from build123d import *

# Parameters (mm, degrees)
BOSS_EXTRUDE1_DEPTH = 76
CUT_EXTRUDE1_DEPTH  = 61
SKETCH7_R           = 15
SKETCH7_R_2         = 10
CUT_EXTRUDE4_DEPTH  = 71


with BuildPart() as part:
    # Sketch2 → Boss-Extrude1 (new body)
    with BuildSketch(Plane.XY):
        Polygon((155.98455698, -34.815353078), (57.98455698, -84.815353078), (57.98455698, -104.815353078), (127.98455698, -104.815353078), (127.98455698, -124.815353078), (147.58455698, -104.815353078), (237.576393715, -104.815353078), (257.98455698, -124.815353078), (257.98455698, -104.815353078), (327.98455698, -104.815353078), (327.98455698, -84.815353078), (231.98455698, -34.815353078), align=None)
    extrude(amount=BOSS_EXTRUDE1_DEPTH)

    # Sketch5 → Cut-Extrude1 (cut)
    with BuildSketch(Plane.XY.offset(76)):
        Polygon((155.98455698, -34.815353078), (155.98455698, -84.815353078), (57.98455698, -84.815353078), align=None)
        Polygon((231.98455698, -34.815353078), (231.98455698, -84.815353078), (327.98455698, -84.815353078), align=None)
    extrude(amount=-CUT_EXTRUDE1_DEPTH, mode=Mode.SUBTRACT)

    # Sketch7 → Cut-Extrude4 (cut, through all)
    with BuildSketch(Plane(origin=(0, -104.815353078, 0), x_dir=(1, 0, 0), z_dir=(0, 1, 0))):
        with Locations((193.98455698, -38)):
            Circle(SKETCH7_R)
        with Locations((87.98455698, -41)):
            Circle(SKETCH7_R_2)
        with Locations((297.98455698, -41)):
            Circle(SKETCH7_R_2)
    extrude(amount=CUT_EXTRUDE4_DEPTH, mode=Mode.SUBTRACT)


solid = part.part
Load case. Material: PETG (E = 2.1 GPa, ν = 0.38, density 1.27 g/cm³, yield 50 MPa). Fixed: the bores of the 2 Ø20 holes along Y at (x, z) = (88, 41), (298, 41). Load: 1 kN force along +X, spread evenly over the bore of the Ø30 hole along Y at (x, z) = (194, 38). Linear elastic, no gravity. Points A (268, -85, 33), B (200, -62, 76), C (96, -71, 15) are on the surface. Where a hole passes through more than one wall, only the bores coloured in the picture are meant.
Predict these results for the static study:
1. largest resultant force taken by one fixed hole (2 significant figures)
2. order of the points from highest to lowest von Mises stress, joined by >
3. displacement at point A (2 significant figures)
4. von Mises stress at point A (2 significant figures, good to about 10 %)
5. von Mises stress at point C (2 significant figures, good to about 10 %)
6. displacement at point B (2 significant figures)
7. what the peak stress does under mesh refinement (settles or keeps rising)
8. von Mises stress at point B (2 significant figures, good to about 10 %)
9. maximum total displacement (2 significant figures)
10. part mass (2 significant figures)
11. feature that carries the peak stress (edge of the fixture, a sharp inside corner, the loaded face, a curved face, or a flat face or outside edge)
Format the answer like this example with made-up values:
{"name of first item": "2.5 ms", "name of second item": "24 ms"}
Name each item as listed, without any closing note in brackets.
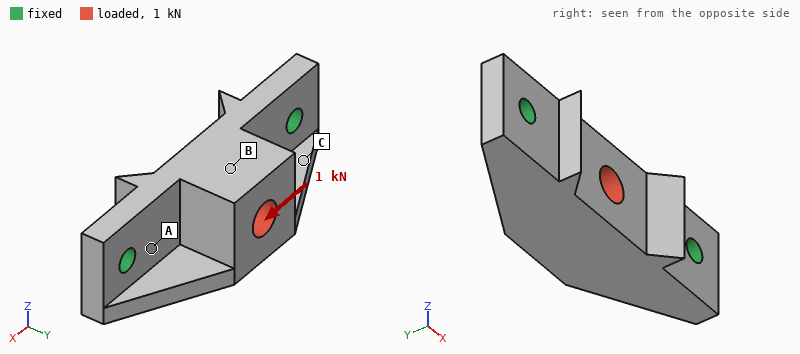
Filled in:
{"largest resultant force taken by one fixed hole": "520 N", "order of the points from highest to lowest von Mises stress, joined by >": "A > C > B", "displacement at point A": "7.8 µm", "von Mises stress at point A": "0.52 MPa", "von Mises stress at point C": "0.34 MPa", "displacement at point B": "28 µm", "what the peak stress does under mesh refinement": "keeps rising", "von Mises stress at point B": "0.13 MPa", "maximum total displacement": "42 µm", "part mass": "940 g", "feature that carries the peak stress": "edge of the fixture"}
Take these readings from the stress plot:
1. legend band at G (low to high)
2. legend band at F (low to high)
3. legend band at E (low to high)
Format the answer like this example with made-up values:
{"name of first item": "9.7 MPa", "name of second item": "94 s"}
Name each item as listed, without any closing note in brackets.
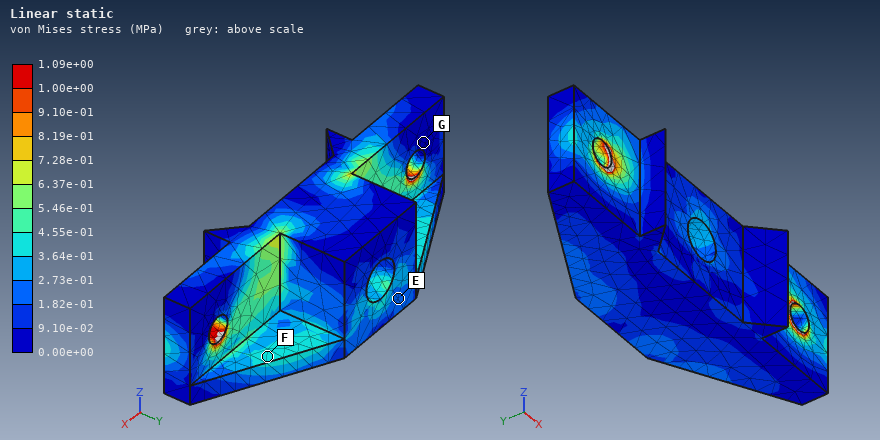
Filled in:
{"legend band at G": "0.00e+00 to 9.10e-02 MPa", "legend band at F": "3.64e-01 to 4.55e-01 MPa", "legend band at E": "1.82e-01 to 2.73e-01 MPa"}
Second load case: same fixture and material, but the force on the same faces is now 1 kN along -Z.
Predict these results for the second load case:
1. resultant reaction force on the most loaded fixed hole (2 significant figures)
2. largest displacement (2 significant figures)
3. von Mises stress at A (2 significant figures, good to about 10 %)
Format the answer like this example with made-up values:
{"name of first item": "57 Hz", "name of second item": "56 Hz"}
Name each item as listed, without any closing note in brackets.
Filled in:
{"resultant reaction force on the most loaded fixed hole": "510 N", "largest displacement": "0.35 mm", "von Mises stress at A": "2.1 MPa"}
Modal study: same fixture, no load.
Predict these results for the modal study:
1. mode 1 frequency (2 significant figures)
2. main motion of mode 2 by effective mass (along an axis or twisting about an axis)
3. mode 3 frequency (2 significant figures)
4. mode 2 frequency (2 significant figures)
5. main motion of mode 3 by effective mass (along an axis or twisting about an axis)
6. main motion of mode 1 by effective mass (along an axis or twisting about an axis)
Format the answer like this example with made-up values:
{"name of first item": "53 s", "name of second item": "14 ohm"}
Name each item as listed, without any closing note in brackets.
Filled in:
{"mode 1 frequency": "410 Hz", "main motion of mode 2 by effective mass": "along Y", "mode 3 frequency": "1000 Hz", "mode 2 frequency": "610 Hz", "main motion of mode 3 by effective mass": "along Z", "main motion of mode 1 by effective mass": "along Z"}
